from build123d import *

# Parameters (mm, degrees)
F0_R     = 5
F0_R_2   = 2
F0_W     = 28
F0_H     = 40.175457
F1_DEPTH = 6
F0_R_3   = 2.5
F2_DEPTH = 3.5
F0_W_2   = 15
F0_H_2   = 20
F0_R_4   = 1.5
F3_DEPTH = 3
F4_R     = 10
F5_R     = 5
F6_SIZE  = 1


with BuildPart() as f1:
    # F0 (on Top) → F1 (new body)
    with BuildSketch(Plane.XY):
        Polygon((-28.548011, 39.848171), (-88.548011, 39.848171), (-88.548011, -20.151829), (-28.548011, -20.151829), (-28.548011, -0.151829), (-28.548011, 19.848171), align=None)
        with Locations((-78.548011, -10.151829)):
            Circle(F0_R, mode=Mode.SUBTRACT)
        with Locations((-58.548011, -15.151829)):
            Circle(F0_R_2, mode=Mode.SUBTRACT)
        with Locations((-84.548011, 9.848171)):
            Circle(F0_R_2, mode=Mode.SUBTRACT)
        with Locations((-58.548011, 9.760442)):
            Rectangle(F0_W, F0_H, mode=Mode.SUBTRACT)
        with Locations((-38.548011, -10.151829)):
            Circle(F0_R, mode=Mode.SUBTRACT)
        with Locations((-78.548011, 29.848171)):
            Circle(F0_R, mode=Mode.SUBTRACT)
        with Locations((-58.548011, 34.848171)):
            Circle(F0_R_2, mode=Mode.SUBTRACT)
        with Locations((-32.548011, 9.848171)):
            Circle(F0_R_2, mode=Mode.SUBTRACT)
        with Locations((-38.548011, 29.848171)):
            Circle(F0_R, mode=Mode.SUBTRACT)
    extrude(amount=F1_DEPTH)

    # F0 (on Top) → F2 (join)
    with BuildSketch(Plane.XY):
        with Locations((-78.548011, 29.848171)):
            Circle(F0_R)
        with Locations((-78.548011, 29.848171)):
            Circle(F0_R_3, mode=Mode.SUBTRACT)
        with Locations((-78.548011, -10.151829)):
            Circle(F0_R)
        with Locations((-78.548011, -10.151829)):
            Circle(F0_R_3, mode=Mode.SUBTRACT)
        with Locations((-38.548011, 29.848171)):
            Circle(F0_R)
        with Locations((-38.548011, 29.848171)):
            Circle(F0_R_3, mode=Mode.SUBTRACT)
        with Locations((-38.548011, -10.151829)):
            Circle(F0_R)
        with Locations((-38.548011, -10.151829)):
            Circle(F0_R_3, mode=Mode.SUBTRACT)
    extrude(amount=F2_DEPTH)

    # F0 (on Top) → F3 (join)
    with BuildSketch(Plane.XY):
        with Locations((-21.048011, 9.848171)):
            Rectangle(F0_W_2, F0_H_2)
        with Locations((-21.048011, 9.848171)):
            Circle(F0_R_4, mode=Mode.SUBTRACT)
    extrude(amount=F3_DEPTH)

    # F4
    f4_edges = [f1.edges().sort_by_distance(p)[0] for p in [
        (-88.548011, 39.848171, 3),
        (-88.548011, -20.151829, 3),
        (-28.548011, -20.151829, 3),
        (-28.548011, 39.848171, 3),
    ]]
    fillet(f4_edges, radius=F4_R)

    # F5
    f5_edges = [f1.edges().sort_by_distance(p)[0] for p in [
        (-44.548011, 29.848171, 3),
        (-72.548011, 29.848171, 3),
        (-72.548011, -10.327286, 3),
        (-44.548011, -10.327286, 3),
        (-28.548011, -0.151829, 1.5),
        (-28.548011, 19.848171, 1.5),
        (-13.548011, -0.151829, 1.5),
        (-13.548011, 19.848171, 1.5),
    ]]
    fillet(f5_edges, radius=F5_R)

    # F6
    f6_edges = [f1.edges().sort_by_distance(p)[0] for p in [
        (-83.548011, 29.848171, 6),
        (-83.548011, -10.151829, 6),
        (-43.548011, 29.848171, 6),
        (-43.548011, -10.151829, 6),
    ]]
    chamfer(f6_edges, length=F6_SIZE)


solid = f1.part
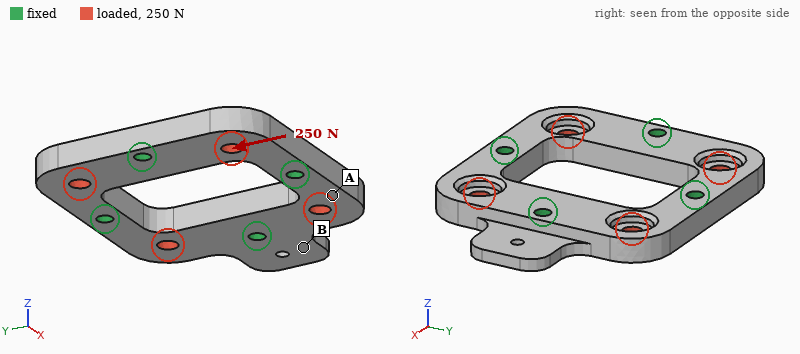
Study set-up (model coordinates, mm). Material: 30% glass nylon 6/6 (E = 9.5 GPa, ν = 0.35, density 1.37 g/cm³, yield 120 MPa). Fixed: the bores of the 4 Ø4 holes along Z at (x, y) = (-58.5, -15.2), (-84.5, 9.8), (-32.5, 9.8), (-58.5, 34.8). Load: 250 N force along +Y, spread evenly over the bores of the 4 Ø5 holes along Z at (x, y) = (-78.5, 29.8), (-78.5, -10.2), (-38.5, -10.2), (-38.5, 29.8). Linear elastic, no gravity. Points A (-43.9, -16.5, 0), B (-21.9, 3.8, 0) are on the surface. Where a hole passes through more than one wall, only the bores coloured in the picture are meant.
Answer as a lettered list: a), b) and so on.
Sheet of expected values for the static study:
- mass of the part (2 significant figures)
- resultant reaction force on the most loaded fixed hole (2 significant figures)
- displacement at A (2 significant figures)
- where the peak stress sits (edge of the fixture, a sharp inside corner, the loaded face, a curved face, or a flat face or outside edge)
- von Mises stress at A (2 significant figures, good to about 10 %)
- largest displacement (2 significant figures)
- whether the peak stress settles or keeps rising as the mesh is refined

a) 19 g
b) 110 N
c) 2.6 µm
d) edge of the fixture
e) 0.76 MPa
f) 4.4 µm
g) keeps rising
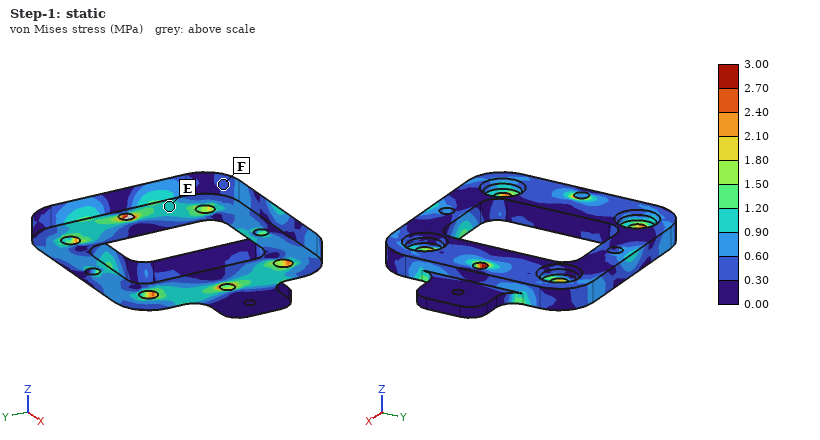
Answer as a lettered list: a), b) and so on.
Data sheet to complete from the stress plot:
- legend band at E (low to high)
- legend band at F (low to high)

a) 0.90 to 1.20 MPa
b) 0.30 to 0.60 MPa
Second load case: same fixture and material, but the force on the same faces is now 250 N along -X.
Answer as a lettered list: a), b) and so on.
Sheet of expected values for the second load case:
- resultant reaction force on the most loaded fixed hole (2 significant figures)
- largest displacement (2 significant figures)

a) 86 N
b) 4.4 µm
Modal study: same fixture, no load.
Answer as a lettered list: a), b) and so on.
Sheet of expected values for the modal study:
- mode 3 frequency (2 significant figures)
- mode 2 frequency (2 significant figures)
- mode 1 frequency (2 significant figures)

a) 5500 Hz
b) 5400 Hz
c) 5000 Hz
